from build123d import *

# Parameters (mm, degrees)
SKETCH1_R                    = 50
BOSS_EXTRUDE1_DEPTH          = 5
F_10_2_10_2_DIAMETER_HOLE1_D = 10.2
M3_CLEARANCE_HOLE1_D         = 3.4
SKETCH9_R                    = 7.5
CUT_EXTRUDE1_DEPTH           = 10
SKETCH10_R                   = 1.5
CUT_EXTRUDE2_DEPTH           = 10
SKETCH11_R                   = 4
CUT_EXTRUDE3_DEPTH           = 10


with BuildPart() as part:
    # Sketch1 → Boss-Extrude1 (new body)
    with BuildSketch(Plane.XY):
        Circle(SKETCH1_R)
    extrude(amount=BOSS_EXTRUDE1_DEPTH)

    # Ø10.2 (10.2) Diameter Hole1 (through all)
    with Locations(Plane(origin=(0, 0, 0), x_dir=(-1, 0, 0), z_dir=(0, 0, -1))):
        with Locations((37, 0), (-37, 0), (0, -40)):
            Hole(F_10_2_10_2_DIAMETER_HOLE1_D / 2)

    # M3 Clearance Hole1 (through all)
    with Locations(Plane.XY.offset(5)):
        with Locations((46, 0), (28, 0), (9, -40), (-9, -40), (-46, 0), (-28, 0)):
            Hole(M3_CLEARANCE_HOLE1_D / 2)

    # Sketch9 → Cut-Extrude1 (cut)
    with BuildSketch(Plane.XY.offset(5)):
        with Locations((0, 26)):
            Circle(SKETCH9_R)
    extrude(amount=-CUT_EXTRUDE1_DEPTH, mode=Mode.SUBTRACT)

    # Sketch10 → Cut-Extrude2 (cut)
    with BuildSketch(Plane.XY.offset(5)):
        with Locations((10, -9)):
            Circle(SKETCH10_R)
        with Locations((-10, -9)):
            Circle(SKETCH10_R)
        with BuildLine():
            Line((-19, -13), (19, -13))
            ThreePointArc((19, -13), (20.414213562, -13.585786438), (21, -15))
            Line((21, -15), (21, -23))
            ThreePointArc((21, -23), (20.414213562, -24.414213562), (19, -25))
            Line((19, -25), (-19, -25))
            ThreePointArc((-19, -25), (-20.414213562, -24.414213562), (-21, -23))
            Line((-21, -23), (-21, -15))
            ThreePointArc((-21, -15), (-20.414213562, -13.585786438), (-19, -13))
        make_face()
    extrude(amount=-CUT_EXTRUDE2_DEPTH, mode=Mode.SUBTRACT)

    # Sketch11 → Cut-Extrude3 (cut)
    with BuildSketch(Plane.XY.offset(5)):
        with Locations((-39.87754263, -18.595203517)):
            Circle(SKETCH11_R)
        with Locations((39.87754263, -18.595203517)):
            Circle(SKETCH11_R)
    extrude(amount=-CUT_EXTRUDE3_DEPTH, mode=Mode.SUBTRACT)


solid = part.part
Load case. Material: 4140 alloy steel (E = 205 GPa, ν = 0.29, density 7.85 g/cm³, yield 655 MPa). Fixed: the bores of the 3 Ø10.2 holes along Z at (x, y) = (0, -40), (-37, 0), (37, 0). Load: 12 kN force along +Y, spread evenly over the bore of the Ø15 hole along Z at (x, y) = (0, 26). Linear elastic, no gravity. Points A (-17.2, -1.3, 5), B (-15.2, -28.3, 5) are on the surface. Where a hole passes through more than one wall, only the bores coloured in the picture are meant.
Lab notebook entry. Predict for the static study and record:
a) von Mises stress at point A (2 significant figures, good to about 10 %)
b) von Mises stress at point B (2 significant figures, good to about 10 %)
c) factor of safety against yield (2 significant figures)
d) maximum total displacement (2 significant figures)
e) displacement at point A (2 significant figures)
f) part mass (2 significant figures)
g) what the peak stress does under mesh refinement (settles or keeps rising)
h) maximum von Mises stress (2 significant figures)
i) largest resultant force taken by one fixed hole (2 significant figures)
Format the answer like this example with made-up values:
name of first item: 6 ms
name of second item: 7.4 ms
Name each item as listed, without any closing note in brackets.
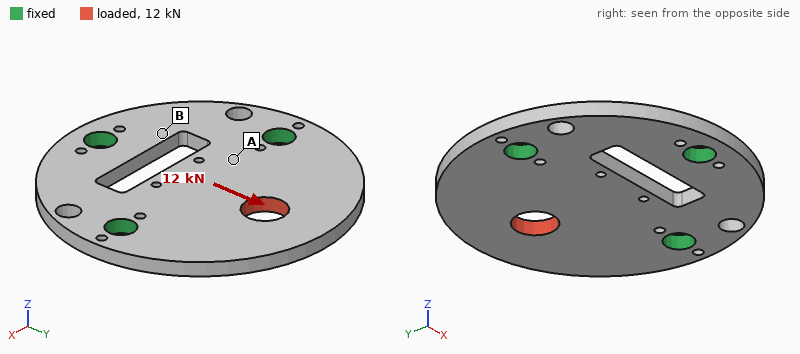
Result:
von Mises stress at point A: 39 MPa
von Mises stress at point B: 11 MPa
factor of safety against yield: 4.7
maximum total displacement: 15 µm
displacement at point A: 6.7 µm
part mass: 270 g
what the peak stress does under mesh refinement: settles
maximum von Mises stress: 140 MPa
largest resultant force taken by one fixed hole: 6.2 kN
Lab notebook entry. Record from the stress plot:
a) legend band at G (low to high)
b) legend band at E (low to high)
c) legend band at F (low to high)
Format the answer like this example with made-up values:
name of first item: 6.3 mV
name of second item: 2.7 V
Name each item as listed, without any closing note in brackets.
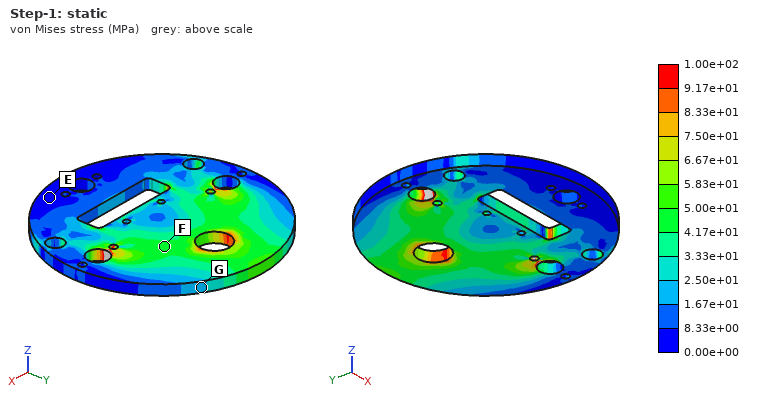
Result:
legend band at G: 1.67e+01 to 2.50e+01 MPa
legend band at E: 0.00e+00 to 8.33e+00 MPa
legend band at F: 4.17e+01 to 5.00e+01 MPa
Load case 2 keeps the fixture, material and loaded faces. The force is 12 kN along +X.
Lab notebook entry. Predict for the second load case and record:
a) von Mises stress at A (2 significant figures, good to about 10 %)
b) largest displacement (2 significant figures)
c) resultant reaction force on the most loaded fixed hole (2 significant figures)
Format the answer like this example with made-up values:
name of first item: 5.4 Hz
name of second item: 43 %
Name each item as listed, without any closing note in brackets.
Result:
von Mises stress at A: 27 MPa
largest displacement: 17 µm
resultant reaction force on the most loaded fixed hole: 7.0 kN
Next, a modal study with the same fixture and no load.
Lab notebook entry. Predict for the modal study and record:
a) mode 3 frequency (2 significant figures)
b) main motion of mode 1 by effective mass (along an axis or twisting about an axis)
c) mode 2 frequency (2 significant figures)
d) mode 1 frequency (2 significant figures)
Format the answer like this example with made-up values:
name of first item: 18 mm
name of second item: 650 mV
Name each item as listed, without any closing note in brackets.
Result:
mode 3 frequency: 5800 Hz
main motion of mode 1 by effective mass: along Z
mode 2 frequency: 4600 Hz
mode 1 frequency: 1900 Hz
